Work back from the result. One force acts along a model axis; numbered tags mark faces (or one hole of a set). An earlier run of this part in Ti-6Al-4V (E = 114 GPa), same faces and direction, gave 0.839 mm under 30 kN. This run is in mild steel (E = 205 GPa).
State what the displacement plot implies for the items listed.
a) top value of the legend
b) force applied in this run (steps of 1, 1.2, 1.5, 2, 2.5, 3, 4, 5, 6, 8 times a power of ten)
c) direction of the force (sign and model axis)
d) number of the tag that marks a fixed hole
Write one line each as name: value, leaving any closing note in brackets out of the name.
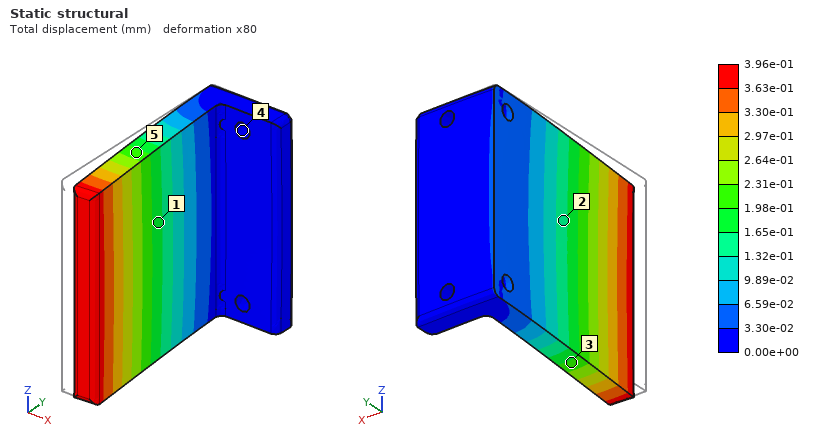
top value of the legend: 3.96e-01 mm
force applied in this run: 25 kN
direction of the force: +X
number of the tag that marks a fixed hole: 4
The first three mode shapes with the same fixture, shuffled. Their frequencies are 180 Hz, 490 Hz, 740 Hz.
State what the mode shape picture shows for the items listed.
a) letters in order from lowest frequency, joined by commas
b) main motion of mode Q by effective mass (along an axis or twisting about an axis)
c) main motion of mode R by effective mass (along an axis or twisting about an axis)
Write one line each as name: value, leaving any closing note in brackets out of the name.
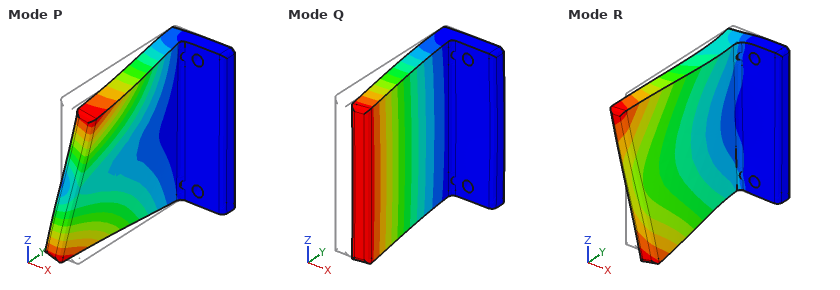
letters in order from lowest frequency, joined by commas: Q, P, R
main motion of mode Q by effective mass: along X
main motion of mode R by effective mass: along Z
